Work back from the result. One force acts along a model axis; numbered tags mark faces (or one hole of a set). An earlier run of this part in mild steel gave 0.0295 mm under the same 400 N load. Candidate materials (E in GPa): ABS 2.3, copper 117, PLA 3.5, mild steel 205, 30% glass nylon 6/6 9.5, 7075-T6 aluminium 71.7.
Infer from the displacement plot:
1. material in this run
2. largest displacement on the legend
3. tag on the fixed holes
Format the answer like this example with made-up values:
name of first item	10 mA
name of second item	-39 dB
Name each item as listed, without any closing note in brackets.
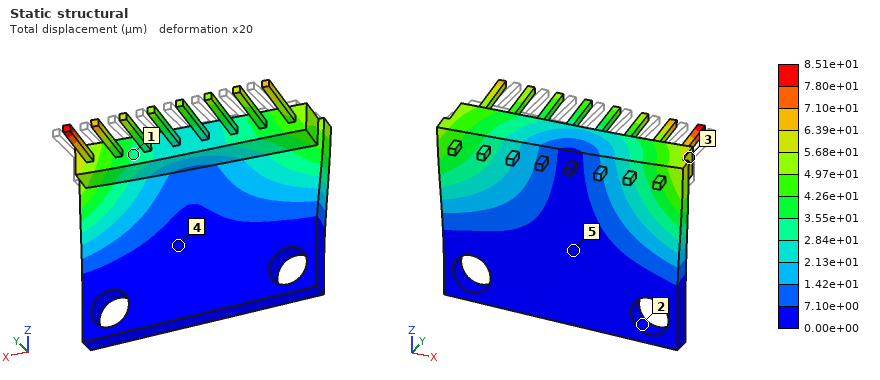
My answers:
material in this run	7075-T6 aluminium
largest displacement on the legend	8.51e+01 µm
tag on the fixed holes	2
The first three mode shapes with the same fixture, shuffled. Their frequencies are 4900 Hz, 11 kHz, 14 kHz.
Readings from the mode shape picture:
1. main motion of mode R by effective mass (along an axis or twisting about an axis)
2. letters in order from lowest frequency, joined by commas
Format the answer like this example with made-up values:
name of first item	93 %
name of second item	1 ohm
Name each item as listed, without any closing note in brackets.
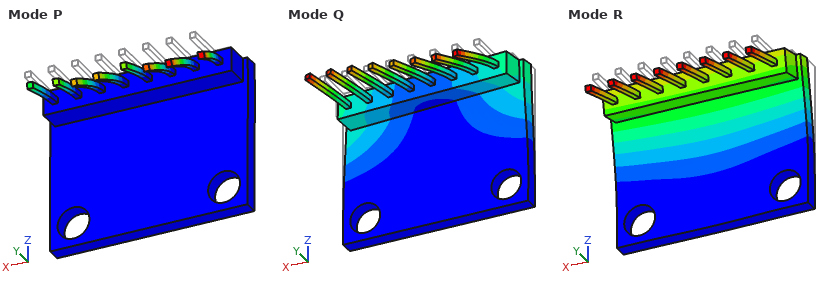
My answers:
main motion of mode R by effective mass	along Y
letters in order from lowest frequency, joined by commas	R, Q, P
